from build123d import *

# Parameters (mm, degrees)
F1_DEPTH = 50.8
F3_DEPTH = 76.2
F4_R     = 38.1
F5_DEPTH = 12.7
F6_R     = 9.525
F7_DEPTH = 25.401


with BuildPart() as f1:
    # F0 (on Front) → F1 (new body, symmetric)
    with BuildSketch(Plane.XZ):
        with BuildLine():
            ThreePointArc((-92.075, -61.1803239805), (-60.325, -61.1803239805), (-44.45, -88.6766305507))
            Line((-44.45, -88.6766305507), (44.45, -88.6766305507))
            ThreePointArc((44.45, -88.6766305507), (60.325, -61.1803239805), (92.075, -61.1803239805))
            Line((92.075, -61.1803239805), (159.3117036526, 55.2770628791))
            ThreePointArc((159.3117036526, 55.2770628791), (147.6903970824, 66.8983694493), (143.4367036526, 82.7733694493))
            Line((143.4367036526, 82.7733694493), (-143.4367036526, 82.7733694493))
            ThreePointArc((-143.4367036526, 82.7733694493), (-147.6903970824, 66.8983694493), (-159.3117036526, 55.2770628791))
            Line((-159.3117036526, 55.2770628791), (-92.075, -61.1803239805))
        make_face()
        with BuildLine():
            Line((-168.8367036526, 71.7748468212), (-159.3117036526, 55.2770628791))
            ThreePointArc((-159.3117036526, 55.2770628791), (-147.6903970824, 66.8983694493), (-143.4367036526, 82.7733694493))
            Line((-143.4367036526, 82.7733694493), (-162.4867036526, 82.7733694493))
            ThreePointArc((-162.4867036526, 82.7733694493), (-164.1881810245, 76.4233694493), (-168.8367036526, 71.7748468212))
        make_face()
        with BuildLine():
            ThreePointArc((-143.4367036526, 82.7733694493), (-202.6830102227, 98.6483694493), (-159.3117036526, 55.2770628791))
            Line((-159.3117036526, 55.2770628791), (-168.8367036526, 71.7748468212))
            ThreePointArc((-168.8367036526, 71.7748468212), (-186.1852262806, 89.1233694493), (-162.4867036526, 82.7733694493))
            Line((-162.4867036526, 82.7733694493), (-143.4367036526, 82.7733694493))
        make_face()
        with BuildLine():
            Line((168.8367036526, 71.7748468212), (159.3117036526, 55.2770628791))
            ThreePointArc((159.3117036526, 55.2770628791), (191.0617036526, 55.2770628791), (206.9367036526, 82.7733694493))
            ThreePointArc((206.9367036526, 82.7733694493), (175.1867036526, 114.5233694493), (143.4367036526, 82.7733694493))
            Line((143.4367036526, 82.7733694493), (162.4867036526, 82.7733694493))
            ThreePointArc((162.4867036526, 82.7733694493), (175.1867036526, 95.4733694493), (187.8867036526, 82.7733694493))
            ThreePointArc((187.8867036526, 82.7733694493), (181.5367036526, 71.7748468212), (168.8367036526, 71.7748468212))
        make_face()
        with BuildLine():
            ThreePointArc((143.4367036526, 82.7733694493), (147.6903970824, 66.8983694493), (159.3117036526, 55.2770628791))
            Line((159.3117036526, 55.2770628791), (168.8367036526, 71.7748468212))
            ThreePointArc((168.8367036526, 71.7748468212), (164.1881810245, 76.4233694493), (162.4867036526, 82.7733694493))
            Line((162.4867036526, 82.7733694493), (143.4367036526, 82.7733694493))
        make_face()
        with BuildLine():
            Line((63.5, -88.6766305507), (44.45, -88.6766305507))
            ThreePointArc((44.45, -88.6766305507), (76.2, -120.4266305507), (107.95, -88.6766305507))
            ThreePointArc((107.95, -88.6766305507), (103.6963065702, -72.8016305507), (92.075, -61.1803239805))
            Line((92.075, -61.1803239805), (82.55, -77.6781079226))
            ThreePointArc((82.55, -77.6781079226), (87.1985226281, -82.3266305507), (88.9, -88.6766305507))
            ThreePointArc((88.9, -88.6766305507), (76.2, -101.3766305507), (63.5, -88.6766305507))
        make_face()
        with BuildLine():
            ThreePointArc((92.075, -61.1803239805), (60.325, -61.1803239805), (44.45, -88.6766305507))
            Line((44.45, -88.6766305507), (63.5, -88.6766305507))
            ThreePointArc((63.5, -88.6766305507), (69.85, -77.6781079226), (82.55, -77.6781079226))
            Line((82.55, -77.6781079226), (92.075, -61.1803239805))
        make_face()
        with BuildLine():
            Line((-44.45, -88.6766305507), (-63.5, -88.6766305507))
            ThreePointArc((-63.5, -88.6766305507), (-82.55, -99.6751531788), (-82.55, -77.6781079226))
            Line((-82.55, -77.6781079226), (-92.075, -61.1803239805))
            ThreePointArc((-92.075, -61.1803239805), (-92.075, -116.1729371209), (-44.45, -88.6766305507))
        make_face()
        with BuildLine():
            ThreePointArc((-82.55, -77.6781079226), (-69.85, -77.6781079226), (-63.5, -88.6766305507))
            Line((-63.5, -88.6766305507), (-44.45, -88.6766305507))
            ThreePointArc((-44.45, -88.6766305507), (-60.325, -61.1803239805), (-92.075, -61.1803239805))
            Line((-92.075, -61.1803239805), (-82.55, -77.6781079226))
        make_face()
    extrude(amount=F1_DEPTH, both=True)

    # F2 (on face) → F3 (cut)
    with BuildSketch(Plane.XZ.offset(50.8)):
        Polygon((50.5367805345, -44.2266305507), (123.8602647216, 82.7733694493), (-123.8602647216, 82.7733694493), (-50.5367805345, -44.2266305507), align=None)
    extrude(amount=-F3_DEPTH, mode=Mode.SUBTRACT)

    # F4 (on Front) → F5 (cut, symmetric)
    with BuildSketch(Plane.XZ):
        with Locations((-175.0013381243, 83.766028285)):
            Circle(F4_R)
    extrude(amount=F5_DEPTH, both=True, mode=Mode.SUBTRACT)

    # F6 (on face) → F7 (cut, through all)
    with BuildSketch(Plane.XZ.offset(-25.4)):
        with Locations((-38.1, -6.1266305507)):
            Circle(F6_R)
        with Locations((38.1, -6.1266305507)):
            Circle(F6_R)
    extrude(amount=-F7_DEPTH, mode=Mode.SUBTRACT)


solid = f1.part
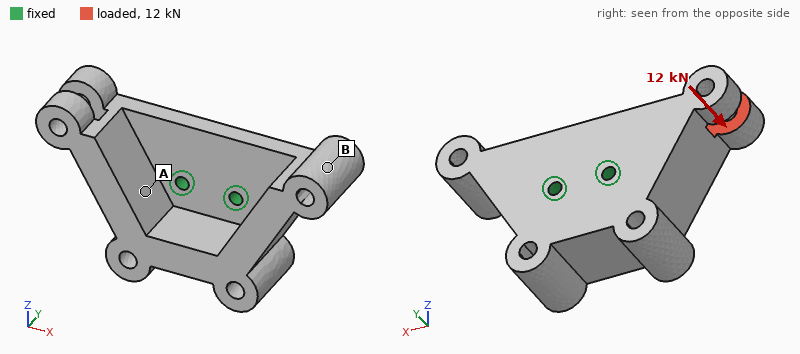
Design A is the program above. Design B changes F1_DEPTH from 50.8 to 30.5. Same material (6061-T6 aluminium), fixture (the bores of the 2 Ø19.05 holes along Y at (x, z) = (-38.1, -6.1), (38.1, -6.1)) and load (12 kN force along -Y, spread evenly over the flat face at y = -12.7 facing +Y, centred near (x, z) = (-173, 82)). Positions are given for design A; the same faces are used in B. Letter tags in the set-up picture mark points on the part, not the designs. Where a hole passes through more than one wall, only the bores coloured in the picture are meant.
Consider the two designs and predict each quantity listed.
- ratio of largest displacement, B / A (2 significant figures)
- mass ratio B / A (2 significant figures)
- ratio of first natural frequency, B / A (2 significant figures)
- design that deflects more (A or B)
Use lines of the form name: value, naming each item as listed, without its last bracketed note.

ratio of largest displacement, B / A: 22
mass ratio B / A: 0.53
ratio of first natural frequency, B / A: 0.22
design that deflects more: B
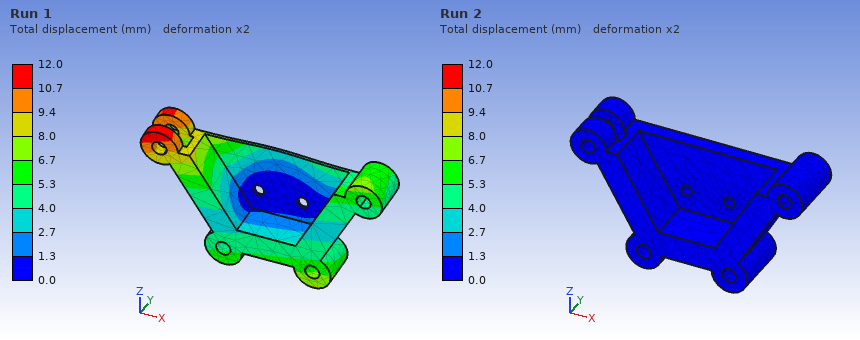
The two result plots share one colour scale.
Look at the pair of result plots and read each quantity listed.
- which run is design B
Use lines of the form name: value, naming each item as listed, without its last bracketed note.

which run is design B: Run 1
